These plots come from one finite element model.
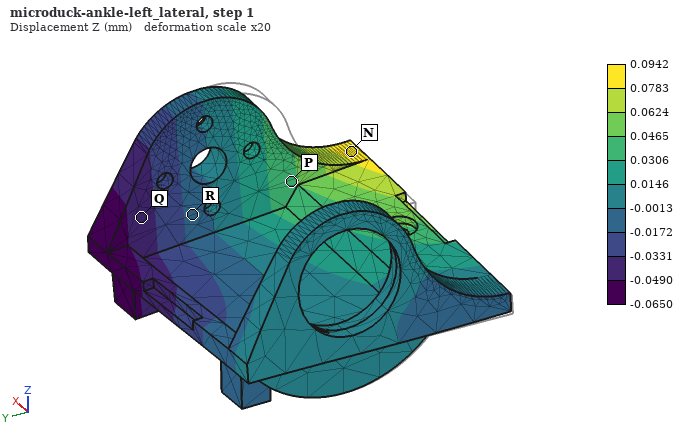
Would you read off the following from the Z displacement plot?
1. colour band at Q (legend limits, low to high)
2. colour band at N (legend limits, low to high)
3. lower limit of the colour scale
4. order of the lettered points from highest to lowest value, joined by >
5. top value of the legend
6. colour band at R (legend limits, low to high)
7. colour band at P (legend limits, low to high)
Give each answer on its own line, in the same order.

-0.0490 to -0.0331 mm
0.0783 to 0.0942 mm
-0.0650 mm
N > P > R > Q
0.0942 mm
-0.0172 to -0.0013 mm
0.0306 to 0.0465 mm
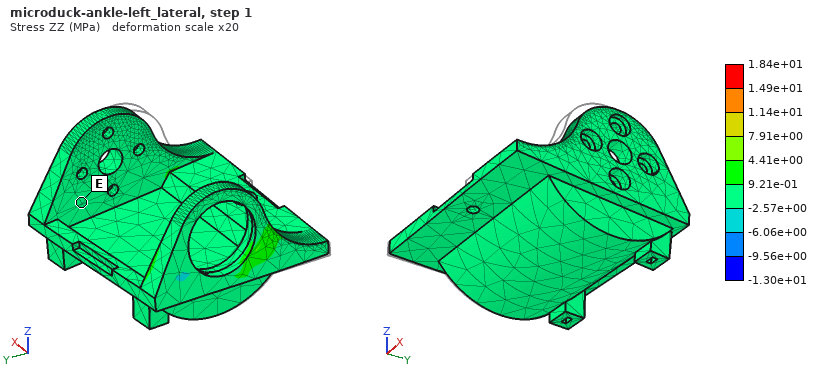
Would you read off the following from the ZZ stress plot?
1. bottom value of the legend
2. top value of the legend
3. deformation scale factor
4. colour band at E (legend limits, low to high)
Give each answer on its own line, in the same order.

-1.30e+01 MPa
1.84e+01 MPa
20
-2.57e+00 to 9.21e-01 MPa
